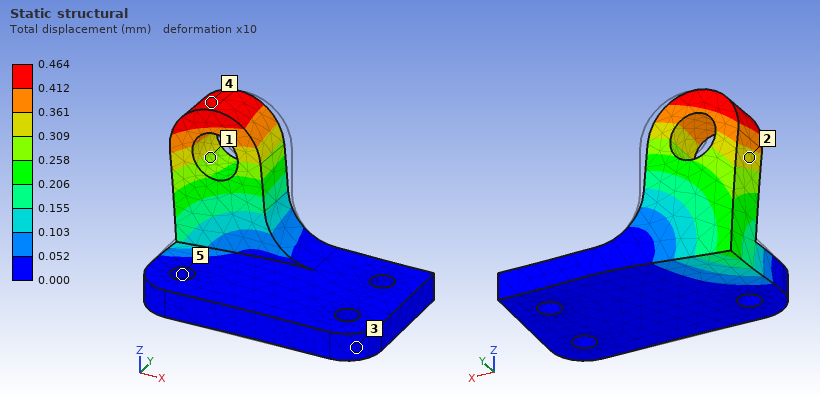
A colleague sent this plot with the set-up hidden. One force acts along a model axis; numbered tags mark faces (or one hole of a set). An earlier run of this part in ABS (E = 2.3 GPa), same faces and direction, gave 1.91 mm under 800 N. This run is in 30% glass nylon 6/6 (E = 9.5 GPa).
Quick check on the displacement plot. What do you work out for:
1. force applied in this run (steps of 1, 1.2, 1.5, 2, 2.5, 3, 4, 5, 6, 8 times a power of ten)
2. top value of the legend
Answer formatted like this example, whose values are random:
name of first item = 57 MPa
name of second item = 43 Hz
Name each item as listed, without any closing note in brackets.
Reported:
force applied in this run = 800 N
top value of the legend = 0.464 mm
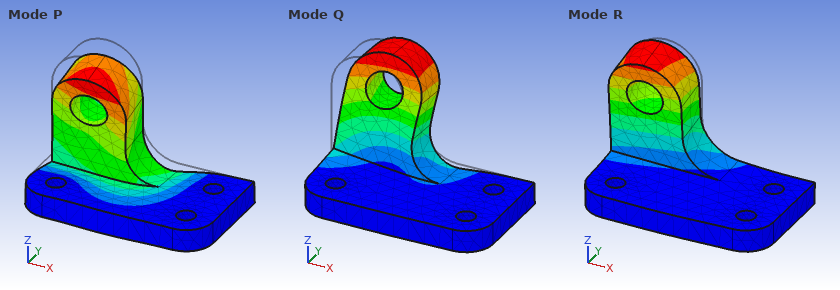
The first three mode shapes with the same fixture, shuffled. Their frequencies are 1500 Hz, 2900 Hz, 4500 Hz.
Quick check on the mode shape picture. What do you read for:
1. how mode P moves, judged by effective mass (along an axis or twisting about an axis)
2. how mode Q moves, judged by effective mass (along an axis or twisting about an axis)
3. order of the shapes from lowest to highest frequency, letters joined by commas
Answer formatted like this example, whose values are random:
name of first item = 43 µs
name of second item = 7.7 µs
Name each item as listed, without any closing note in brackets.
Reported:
how mode P moves, judged by effective mass = along Z
how mode Q moves, judged by effective mass = along X
order of the shapes from lowest to highest frequency, letters joined by commas = R, Q, P
